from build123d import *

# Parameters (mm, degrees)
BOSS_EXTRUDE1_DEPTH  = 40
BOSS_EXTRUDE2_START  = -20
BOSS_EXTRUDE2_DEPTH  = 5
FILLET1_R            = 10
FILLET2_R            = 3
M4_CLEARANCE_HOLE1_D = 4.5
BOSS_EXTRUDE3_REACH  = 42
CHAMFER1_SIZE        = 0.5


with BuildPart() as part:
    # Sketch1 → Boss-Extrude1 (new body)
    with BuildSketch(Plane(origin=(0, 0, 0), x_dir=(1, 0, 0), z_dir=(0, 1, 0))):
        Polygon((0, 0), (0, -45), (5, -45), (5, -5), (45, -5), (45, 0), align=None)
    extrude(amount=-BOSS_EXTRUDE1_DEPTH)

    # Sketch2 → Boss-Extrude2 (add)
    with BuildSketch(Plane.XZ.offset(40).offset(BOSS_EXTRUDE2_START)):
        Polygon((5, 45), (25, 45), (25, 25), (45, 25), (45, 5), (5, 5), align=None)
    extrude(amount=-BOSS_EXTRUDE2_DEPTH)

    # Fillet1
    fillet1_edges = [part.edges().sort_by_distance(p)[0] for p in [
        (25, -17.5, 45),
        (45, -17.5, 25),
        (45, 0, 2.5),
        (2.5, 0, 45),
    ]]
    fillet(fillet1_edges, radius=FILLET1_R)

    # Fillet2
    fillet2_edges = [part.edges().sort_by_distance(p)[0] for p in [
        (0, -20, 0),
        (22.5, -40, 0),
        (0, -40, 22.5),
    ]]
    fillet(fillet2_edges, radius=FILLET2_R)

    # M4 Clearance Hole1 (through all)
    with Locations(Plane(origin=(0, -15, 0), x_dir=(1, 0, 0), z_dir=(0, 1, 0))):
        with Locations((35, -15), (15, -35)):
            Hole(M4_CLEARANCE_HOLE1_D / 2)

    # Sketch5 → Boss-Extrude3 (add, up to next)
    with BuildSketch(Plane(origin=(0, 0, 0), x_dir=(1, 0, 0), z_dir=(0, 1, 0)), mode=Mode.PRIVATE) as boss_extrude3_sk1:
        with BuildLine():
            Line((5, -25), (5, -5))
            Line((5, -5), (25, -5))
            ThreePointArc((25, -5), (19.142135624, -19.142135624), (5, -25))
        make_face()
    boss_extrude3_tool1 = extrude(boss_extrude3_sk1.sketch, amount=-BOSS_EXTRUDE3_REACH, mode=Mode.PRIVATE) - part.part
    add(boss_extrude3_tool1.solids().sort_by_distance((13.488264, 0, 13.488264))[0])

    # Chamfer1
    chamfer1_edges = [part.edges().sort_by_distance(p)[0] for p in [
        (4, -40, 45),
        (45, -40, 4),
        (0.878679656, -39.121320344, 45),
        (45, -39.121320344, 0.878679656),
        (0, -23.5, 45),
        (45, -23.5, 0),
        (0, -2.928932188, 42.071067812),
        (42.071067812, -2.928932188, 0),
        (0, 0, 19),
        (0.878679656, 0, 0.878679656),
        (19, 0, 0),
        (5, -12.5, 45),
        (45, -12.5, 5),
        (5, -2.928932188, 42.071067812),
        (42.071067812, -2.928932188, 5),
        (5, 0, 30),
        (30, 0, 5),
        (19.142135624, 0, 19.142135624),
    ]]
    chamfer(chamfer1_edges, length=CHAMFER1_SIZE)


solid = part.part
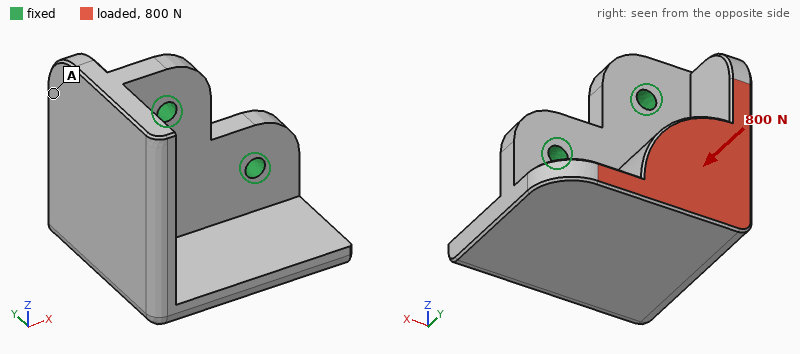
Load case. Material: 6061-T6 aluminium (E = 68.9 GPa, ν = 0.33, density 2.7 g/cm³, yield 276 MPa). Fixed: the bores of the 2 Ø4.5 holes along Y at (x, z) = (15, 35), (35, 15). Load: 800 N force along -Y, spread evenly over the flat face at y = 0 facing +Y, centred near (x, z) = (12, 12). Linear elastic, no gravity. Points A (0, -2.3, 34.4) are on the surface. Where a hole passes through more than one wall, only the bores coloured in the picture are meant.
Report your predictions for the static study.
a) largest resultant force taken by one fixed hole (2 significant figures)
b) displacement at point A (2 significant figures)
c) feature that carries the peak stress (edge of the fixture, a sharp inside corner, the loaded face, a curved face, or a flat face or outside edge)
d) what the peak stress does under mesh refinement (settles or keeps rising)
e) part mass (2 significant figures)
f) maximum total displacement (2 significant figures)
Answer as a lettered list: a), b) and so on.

a) 400 N
b) 0.046 mm
c) edge of the fixture
d) keeps rising
e) 72 g
f) 0.10 mm
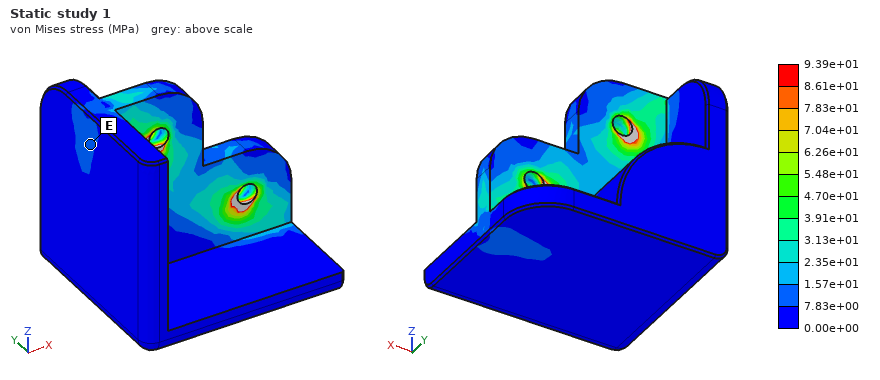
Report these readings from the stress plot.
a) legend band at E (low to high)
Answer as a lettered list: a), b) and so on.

a) 7.83e+00 to 1.57e+01 MPa
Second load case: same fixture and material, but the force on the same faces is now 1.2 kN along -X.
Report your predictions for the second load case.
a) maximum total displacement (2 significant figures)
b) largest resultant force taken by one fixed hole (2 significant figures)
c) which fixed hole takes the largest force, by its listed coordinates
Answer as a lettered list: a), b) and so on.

a) 0.14 mm
b) 1.1 kN
c) (35, 15)
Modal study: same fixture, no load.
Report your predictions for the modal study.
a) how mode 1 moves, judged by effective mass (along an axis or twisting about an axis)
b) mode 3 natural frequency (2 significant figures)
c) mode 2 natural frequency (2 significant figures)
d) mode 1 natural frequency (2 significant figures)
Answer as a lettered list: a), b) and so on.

a) along Y
b) 9100 Hz
c) 5600 Hz
d) 2200 Hz
